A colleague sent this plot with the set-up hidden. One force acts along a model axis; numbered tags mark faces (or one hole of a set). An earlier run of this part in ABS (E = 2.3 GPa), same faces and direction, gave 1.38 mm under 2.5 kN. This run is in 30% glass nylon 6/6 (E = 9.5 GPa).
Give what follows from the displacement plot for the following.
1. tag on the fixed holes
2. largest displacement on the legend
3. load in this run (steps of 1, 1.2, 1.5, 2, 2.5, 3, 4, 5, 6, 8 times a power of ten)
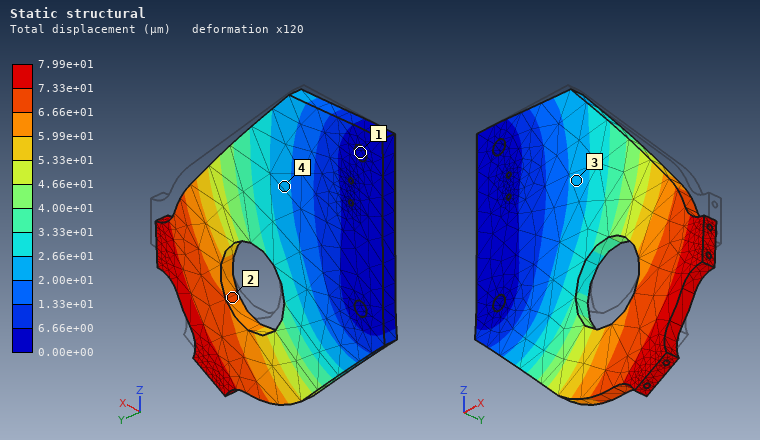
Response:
1
7.99e+01 µm
600 N
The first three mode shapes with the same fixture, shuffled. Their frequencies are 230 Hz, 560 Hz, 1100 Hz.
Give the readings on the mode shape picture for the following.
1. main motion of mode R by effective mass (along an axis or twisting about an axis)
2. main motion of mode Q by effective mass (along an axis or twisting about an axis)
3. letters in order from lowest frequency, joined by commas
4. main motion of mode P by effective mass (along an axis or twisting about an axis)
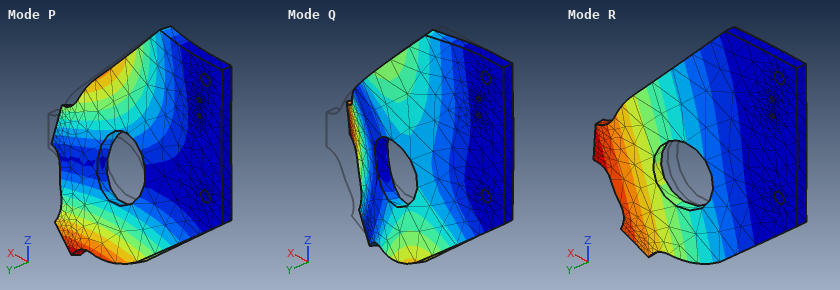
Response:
along Y
along Y
R, P, Q
twisting about X
